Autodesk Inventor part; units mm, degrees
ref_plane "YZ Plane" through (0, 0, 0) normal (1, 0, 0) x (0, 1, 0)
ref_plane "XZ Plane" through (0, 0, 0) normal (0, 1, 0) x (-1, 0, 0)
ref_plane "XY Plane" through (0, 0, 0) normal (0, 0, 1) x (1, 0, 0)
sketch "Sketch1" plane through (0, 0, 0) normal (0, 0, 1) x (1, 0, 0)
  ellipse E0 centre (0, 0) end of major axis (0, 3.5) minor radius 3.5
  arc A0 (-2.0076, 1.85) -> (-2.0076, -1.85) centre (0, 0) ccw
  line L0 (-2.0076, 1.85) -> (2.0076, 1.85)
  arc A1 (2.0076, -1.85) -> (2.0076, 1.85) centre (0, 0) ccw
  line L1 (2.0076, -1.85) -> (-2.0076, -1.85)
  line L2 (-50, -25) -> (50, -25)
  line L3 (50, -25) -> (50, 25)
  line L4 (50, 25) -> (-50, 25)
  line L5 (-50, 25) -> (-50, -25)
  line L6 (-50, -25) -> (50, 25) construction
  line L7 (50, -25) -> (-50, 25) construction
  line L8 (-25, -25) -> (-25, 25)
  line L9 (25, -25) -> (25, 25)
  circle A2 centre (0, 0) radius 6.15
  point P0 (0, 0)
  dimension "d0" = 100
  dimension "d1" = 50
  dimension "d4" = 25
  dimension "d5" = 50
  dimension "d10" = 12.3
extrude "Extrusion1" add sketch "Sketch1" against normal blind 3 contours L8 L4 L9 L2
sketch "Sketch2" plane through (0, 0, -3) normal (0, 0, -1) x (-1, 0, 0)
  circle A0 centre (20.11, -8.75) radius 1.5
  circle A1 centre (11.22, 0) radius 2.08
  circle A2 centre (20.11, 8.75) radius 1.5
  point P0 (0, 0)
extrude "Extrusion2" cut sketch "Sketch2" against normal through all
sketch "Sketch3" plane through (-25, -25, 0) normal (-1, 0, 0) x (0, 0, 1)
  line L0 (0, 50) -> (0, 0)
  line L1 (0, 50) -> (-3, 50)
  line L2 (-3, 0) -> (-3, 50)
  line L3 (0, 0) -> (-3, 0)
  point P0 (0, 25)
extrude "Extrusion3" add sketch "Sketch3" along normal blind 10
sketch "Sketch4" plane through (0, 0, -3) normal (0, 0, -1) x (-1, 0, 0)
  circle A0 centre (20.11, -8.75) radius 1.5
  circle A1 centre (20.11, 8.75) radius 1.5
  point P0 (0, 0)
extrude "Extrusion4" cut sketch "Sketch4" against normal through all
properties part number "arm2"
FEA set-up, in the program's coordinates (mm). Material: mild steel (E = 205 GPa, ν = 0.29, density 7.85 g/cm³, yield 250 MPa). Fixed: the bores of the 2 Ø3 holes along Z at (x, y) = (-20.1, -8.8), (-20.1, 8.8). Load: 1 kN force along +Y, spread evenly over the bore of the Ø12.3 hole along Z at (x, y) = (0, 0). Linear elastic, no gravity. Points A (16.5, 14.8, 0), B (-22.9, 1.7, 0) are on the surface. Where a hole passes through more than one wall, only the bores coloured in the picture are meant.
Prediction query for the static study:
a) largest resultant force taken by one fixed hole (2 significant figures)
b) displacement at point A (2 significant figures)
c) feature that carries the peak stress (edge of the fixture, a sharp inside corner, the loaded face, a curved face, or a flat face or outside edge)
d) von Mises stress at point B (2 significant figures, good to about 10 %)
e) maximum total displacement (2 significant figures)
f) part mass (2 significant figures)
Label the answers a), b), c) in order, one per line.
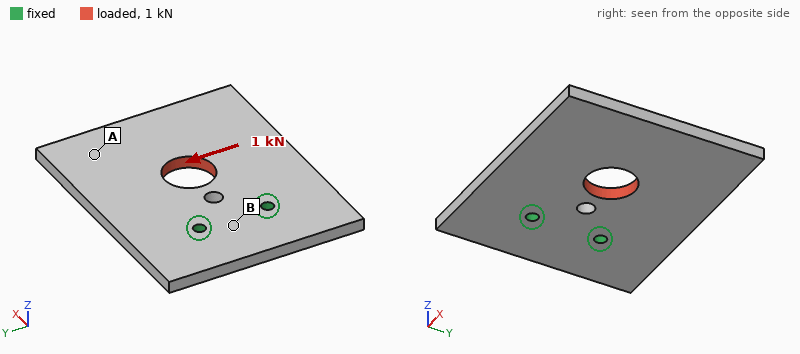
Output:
a) 1.1 kN
b) 9.8 µm
c) edge of the fixture
d) 14 MPa
e) 12 µm
f) 67 g
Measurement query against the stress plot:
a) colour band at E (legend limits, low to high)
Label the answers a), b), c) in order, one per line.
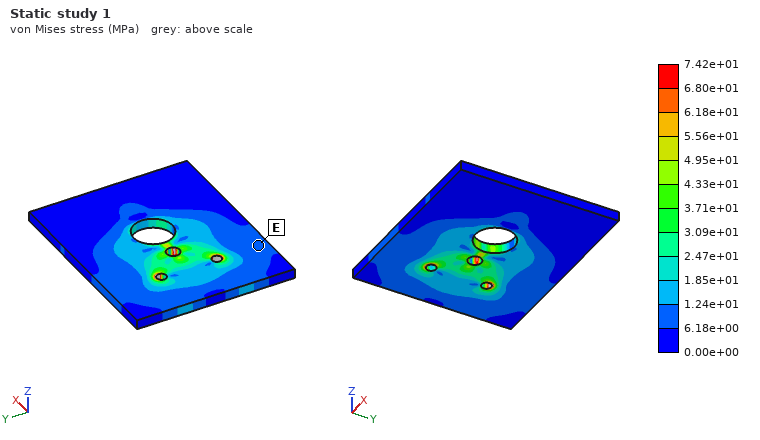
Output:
a) 6.18e+00 to 1.24e+01 MPa
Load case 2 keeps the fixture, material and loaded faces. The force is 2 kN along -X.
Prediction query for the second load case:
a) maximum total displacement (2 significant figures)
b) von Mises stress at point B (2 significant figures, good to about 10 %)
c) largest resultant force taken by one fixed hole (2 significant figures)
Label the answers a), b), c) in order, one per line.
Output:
a) 3.7 µm
b) 6.1 MPa
c) 1.0 kN
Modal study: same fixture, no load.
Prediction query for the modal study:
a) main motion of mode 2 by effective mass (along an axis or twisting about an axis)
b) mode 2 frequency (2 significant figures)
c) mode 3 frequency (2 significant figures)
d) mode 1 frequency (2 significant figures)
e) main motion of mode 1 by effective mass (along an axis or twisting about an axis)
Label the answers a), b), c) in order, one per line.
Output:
a) twisting about X
b) 2300 Hz
c) 5800 Hz
d) 1100 Hz
e) along Z
